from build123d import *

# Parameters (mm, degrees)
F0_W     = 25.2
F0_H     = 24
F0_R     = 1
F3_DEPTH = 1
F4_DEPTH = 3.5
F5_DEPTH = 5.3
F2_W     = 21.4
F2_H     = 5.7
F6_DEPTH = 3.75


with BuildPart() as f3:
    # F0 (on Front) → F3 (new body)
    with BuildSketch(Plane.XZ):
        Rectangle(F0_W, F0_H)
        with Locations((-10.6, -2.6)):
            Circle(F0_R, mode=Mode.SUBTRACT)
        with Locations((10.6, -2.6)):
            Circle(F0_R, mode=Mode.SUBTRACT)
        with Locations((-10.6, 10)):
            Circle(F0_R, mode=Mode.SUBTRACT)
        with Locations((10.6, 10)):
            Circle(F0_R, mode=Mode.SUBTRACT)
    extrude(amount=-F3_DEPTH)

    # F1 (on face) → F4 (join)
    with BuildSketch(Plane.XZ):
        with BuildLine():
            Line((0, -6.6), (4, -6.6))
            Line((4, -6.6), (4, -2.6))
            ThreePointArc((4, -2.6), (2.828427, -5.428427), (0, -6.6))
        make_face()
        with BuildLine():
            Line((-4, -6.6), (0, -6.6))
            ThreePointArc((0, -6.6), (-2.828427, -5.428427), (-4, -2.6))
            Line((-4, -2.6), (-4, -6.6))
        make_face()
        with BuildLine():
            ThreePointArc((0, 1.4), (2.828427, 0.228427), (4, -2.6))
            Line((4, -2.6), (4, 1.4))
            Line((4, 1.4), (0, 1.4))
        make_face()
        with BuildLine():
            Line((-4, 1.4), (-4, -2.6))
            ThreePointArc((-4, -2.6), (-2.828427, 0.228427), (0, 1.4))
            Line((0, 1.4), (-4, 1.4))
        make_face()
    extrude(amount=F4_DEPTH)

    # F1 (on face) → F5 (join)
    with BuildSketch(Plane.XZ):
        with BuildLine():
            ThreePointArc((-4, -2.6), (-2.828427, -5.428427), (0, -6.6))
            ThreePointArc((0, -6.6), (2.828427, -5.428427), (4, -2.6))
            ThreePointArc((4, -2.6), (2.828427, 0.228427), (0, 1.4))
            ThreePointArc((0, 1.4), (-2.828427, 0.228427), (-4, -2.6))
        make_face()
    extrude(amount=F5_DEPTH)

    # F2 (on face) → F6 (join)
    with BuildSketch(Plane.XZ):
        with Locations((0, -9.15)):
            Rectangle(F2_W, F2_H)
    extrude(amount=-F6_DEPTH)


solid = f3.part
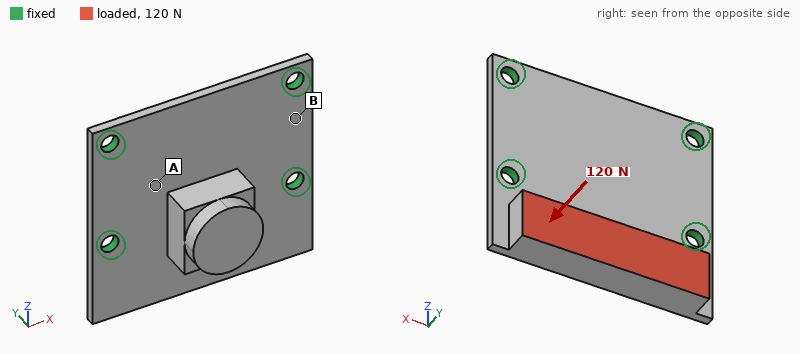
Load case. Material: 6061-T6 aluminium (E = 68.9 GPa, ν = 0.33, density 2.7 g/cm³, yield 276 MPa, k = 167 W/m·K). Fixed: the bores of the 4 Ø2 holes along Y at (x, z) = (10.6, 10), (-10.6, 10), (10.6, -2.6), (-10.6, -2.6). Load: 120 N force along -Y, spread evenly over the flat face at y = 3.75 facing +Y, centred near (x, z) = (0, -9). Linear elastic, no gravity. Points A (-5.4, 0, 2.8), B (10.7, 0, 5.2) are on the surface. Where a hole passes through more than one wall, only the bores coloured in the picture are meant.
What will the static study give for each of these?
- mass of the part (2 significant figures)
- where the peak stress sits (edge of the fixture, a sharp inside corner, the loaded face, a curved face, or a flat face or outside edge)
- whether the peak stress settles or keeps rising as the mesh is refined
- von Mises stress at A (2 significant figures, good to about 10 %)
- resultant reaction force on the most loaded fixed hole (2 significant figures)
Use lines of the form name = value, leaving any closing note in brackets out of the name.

mass of the part = 3.4 g
where the peak stress sits = edge of the fixture
whether the peak stress settles or keeps rising as the mesh is refined = keeps rising
von Mises stress at A = 32 MPa
resultant reaction force on the most loaded fixed hole = 74 N
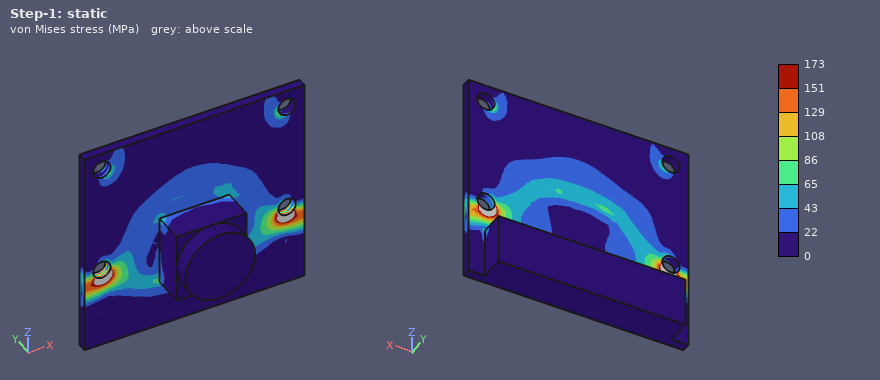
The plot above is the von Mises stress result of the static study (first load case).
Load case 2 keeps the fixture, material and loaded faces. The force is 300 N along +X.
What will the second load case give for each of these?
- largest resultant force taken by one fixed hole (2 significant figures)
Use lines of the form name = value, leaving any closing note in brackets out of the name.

largest resultant force taken by one fixed hole = 170 N
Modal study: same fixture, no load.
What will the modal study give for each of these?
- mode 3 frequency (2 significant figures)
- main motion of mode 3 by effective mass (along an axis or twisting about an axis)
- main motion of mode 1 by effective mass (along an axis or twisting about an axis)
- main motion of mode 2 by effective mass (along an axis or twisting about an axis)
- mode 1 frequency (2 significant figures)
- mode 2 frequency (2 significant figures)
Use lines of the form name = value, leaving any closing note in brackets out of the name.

mode 3 frequency = 17 kHz
main motion of mode 3 by effective mass = twisting about Z
main motion of mode 1 by effective mass = along Y
main motion of mode 2 by effective mass = along Y
mode 1 frequency = 5600 Hz
mode 2 frequency = 11 kHz
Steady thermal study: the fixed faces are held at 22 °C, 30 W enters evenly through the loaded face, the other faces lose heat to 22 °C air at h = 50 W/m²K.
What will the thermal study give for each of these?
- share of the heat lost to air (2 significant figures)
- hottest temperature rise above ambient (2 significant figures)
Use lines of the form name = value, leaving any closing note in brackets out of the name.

share of the heat lost to air = 5.7 %
hottest temperature rise above ambient = 51 K
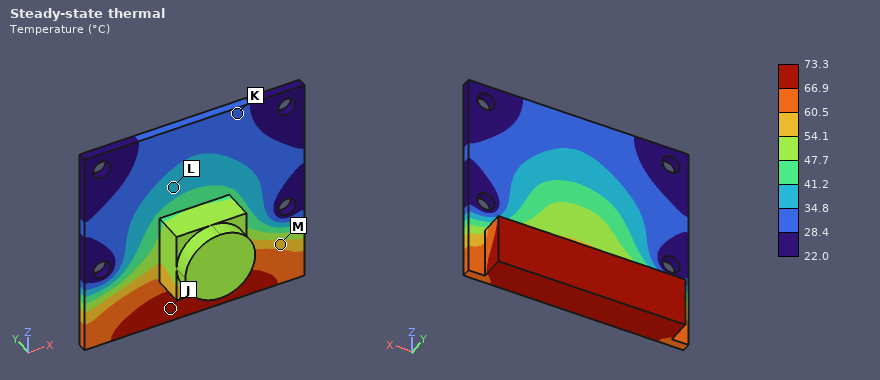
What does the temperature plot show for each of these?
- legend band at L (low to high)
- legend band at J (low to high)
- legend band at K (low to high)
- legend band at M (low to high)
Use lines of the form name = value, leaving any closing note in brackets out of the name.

legend band at L = 34.8 to 41.2 °C
legend band at J = 66.9 to 73.3 °C
legend band at K = 28.4 to 34.8 °C
legend band at M = 54.1 to 60.5 °C
